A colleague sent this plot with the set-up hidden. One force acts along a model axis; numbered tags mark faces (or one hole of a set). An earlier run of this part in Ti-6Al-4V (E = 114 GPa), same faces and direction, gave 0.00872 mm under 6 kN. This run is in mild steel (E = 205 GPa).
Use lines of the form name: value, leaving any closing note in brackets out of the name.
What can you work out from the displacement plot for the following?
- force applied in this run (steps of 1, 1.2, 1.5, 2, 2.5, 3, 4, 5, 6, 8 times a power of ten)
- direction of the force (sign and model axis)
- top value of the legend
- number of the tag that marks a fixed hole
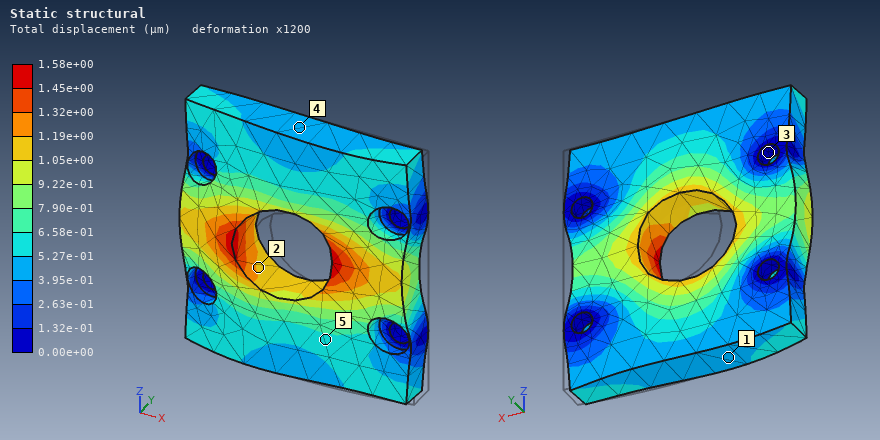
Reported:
force applied in this run: 2 kN
direction of the force: -X
top value of the legend: 1.58e+00 µm
number of the tag that marks a fixed hole: 3
